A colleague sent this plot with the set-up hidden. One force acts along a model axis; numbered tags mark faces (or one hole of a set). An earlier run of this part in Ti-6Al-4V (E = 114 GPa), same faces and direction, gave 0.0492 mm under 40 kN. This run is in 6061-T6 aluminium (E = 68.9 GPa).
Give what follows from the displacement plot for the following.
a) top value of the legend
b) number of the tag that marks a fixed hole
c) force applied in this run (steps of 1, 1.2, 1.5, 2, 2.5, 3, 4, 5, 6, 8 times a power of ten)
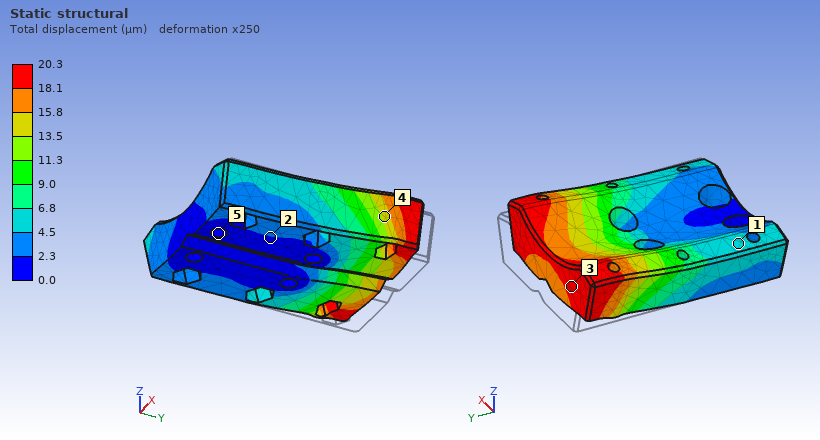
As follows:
20.3 µm
5
10 kN
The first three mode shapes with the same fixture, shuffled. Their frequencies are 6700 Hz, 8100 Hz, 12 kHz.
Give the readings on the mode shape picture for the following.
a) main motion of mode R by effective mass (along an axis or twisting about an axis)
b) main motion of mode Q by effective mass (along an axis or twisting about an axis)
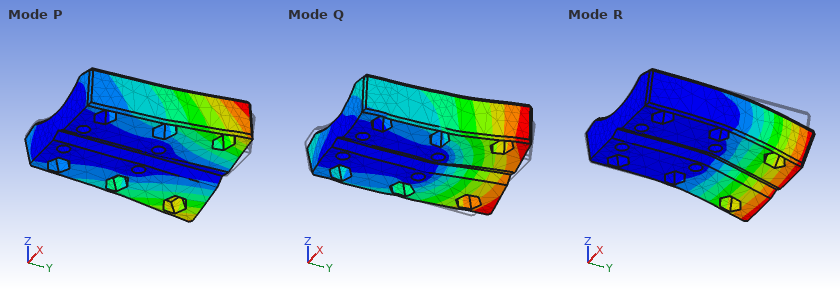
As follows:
along Z
along X
